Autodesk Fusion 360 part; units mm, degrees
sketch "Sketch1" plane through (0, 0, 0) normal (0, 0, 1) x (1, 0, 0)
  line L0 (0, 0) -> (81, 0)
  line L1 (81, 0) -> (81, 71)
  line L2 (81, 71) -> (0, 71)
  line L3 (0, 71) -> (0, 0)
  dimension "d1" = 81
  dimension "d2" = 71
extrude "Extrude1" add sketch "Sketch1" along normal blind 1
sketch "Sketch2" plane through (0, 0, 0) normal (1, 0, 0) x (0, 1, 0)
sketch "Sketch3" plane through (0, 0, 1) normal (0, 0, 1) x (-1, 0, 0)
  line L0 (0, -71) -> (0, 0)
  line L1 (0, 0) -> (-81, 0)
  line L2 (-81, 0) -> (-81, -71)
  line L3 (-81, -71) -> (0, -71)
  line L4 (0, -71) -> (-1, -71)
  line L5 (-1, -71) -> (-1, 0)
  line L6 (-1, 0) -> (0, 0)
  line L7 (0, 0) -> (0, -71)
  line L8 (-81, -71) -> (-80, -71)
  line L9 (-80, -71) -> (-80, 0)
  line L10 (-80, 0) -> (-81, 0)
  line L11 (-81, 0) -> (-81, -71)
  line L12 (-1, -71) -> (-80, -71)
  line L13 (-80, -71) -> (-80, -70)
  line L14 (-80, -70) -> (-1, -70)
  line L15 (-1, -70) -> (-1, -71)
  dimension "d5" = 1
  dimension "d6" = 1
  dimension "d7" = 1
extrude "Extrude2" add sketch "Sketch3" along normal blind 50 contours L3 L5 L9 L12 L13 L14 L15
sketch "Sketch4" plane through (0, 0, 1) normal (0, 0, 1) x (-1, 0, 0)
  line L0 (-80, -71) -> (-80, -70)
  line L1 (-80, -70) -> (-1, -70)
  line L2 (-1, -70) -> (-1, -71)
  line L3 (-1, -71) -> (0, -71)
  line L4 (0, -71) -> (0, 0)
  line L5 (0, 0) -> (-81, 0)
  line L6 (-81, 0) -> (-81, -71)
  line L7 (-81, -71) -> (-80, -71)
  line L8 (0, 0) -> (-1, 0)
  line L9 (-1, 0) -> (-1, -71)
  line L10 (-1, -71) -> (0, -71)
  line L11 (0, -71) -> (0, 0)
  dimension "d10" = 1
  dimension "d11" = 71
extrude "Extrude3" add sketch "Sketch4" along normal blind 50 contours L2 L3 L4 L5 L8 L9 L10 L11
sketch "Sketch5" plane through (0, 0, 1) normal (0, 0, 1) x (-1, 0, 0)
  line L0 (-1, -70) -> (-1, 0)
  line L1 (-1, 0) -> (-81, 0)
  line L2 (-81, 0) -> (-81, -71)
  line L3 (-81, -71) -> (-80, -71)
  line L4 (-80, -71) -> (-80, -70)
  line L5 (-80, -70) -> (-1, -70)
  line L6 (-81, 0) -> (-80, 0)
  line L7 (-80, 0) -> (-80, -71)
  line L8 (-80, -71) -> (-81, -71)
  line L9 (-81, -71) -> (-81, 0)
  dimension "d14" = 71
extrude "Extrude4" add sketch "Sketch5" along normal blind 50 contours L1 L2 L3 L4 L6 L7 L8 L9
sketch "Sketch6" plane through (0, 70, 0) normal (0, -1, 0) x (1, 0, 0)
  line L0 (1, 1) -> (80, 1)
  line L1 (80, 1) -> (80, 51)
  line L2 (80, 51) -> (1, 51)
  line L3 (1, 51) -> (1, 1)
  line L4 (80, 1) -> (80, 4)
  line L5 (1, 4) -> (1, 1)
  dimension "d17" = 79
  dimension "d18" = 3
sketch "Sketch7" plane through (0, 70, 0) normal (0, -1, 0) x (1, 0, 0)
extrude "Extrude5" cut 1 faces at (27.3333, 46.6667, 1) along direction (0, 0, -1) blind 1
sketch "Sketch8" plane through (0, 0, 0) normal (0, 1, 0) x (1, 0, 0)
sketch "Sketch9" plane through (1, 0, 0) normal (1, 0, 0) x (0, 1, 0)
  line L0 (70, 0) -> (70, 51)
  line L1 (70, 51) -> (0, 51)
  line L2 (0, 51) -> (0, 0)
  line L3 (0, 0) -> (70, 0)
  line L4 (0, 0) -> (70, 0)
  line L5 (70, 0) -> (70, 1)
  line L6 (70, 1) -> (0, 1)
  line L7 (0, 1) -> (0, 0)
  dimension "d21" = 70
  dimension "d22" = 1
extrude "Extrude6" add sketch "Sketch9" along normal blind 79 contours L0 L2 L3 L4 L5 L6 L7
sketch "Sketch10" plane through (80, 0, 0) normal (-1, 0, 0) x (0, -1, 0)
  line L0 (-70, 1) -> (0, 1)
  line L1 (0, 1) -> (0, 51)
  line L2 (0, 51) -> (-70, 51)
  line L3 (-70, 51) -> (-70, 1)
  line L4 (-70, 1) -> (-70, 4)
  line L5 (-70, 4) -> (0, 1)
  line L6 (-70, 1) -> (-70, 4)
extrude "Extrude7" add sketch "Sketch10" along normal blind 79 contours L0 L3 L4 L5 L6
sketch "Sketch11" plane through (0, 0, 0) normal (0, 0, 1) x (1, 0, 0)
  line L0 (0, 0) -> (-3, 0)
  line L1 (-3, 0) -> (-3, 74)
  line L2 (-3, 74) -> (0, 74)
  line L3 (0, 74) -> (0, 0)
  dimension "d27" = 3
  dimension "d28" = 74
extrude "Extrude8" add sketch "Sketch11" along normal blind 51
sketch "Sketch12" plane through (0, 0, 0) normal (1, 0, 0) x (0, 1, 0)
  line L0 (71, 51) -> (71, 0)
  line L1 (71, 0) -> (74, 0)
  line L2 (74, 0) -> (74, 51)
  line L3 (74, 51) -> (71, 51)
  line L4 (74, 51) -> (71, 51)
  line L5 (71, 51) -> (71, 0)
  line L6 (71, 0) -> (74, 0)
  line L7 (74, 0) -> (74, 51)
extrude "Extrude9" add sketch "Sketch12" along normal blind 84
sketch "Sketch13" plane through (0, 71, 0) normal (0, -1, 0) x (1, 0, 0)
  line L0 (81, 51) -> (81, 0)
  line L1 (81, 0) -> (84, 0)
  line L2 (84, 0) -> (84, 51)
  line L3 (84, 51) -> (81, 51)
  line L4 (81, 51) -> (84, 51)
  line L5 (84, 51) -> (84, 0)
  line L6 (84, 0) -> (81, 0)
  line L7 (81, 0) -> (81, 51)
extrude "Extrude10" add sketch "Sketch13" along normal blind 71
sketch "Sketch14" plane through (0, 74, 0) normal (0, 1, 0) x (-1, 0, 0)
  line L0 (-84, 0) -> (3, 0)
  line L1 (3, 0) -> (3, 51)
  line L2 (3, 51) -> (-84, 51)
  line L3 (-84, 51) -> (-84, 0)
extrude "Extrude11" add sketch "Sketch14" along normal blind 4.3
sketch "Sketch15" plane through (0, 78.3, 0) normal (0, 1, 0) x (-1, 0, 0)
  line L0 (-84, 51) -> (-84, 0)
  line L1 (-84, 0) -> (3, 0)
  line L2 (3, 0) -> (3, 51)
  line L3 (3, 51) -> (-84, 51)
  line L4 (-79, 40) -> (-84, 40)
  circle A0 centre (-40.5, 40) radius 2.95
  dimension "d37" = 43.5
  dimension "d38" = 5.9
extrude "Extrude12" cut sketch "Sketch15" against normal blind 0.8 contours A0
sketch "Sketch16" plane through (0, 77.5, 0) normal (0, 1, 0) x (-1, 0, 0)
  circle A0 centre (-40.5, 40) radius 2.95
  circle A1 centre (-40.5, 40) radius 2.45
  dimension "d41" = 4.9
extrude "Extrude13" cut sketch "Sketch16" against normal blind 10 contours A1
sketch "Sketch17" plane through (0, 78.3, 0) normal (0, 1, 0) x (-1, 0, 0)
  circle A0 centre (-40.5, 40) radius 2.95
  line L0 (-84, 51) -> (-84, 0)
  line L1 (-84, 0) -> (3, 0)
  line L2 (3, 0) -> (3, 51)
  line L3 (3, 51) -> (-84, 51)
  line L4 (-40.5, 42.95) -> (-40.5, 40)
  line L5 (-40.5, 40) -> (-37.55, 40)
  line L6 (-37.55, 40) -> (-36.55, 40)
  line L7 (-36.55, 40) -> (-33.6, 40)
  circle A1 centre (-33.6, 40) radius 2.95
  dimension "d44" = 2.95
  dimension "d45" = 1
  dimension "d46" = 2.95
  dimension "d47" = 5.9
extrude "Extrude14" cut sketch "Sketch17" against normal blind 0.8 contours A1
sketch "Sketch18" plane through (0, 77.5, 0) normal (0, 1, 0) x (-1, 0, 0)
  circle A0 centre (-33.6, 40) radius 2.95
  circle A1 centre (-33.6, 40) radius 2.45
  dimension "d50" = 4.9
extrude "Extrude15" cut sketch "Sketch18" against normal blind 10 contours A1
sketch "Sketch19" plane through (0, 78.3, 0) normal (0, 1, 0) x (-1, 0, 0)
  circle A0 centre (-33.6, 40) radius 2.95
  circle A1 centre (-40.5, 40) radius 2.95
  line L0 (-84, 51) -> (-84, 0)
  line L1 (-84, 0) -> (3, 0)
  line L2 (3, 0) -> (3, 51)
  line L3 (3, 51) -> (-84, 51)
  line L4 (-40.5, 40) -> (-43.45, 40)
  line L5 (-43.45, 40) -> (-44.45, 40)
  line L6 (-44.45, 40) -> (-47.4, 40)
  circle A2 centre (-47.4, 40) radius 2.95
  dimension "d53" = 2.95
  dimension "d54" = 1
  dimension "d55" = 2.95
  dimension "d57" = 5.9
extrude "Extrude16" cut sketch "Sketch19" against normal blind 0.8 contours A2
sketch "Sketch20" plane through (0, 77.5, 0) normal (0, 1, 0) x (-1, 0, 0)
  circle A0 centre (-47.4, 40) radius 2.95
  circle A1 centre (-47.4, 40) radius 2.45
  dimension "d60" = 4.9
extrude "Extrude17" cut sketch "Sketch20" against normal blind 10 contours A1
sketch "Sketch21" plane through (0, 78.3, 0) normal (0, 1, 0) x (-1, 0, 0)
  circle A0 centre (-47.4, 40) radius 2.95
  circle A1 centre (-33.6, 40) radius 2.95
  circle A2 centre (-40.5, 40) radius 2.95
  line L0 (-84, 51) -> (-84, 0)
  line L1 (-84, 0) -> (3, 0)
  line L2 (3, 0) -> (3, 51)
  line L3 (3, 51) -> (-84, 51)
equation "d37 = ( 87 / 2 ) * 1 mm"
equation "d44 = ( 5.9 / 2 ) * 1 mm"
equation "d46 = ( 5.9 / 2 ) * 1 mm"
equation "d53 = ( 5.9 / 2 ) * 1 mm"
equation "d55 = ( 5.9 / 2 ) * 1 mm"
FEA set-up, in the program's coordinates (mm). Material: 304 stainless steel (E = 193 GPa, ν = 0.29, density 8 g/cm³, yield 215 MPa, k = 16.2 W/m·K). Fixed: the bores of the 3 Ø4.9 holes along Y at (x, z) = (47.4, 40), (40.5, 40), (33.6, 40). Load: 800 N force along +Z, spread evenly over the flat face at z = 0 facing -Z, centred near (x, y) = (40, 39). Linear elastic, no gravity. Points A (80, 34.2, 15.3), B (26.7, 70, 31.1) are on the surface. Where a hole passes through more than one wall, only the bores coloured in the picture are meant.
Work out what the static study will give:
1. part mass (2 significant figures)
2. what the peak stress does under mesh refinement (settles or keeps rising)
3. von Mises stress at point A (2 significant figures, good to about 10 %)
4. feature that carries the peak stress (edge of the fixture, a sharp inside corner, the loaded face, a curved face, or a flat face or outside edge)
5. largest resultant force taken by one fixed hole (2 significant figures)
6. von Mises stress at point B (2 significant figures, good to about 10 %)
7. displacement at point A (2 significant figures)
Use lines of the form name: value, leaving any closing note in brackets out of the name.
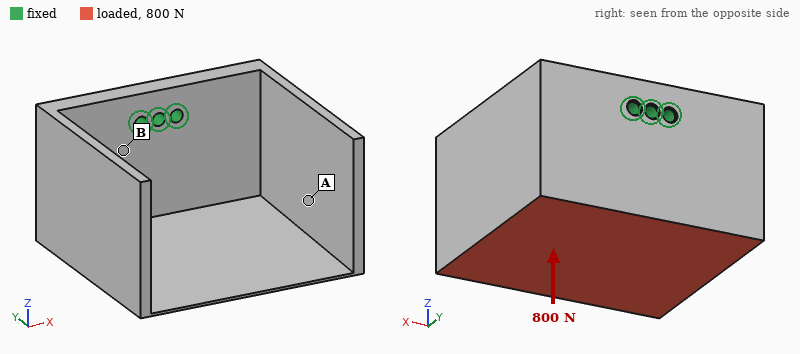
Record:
part mass: 630 g
what the peak stress does under mesh refinement: keeps rising
von Mises stress at point A: 13 MPa
feature that carries the peak stress: edge of the fixture
largest resultant force taken by one fixed hole: 390 N
von Mises stress at point B: 28 MPa
displacement at point A: 0.046 mm
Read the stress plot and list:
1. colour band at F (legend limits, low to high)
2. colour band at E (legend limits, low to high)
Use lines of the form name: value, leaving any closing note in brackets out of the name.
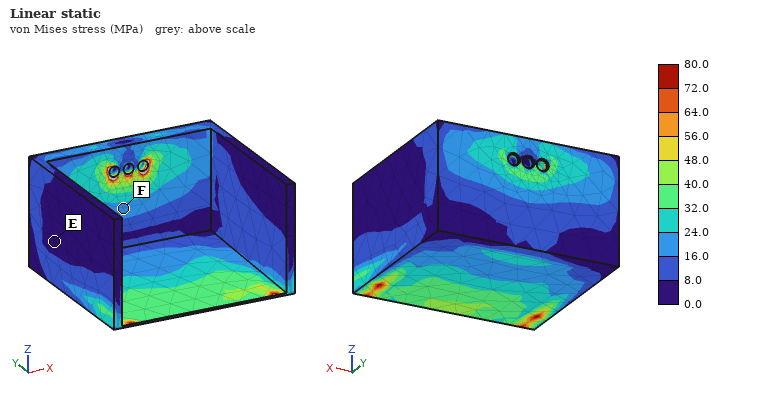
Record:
colour band at F: 16.0 to 24.0 MPa
colour band at E: 0.0 to 8.0 MPa
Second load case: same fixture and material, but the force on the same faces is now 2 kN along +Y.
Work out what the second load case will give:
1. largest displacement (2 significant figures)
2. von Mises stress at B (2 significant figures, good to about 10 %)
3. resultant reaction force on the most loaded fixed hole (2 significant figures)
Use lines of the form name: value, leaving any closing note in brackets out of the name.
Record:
largest displacement: 0.20 mm
von Mises stress at B: 63 MPa
resultant reaction force on the most loaded fixed hole: 720 N
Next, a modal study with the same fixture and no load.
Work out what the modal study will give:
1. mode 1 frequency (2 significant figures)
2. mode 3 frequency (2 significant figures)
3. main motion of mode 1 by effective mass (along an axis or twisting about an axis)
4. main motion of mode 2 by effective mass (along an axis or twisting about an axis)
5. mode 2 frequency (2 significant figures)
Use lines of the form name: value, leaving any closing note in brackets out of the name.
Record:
mode 1 frequency: 760 Hz
mode 3 frequency: 1200 Hz
main motion of mode 1 by effective mass: along X
main motion of mode 2 by effective mass: along Z
mode 2 frequency: 900 Hz
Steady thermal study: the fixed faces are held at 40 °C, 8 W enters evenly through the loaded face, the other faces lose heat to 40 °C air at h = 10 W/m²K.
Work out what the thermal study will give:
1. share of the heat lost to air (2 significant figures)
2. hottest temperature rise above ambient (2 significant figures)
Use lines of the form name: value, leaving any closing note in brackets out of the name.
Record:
share of the heat lost to air: 57 %
hottest temperature rise above ambient: 39 K
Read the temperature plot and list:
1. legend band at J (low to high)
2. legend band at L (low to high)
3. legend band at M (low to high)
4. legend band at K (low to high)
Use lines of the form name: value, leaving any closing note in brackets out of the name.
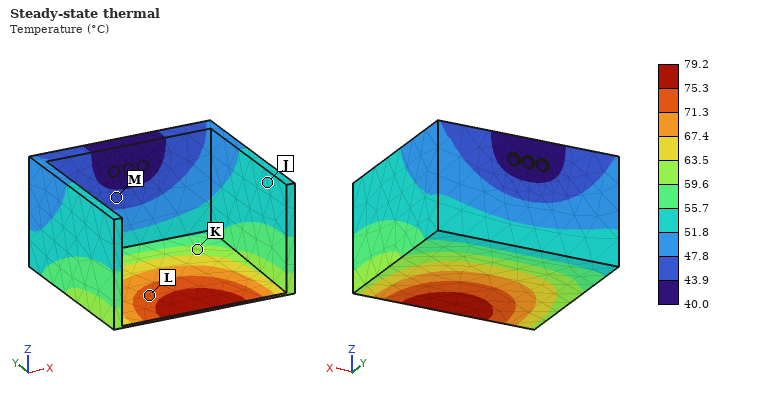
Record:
legend band at J: 51.8 to 55.7 °C
legend band at L: 71.3 to 75.3 °C
legend band at M: 43.9 to 47.8 °C
legend band at K: 59.6 to 63.5 °C
